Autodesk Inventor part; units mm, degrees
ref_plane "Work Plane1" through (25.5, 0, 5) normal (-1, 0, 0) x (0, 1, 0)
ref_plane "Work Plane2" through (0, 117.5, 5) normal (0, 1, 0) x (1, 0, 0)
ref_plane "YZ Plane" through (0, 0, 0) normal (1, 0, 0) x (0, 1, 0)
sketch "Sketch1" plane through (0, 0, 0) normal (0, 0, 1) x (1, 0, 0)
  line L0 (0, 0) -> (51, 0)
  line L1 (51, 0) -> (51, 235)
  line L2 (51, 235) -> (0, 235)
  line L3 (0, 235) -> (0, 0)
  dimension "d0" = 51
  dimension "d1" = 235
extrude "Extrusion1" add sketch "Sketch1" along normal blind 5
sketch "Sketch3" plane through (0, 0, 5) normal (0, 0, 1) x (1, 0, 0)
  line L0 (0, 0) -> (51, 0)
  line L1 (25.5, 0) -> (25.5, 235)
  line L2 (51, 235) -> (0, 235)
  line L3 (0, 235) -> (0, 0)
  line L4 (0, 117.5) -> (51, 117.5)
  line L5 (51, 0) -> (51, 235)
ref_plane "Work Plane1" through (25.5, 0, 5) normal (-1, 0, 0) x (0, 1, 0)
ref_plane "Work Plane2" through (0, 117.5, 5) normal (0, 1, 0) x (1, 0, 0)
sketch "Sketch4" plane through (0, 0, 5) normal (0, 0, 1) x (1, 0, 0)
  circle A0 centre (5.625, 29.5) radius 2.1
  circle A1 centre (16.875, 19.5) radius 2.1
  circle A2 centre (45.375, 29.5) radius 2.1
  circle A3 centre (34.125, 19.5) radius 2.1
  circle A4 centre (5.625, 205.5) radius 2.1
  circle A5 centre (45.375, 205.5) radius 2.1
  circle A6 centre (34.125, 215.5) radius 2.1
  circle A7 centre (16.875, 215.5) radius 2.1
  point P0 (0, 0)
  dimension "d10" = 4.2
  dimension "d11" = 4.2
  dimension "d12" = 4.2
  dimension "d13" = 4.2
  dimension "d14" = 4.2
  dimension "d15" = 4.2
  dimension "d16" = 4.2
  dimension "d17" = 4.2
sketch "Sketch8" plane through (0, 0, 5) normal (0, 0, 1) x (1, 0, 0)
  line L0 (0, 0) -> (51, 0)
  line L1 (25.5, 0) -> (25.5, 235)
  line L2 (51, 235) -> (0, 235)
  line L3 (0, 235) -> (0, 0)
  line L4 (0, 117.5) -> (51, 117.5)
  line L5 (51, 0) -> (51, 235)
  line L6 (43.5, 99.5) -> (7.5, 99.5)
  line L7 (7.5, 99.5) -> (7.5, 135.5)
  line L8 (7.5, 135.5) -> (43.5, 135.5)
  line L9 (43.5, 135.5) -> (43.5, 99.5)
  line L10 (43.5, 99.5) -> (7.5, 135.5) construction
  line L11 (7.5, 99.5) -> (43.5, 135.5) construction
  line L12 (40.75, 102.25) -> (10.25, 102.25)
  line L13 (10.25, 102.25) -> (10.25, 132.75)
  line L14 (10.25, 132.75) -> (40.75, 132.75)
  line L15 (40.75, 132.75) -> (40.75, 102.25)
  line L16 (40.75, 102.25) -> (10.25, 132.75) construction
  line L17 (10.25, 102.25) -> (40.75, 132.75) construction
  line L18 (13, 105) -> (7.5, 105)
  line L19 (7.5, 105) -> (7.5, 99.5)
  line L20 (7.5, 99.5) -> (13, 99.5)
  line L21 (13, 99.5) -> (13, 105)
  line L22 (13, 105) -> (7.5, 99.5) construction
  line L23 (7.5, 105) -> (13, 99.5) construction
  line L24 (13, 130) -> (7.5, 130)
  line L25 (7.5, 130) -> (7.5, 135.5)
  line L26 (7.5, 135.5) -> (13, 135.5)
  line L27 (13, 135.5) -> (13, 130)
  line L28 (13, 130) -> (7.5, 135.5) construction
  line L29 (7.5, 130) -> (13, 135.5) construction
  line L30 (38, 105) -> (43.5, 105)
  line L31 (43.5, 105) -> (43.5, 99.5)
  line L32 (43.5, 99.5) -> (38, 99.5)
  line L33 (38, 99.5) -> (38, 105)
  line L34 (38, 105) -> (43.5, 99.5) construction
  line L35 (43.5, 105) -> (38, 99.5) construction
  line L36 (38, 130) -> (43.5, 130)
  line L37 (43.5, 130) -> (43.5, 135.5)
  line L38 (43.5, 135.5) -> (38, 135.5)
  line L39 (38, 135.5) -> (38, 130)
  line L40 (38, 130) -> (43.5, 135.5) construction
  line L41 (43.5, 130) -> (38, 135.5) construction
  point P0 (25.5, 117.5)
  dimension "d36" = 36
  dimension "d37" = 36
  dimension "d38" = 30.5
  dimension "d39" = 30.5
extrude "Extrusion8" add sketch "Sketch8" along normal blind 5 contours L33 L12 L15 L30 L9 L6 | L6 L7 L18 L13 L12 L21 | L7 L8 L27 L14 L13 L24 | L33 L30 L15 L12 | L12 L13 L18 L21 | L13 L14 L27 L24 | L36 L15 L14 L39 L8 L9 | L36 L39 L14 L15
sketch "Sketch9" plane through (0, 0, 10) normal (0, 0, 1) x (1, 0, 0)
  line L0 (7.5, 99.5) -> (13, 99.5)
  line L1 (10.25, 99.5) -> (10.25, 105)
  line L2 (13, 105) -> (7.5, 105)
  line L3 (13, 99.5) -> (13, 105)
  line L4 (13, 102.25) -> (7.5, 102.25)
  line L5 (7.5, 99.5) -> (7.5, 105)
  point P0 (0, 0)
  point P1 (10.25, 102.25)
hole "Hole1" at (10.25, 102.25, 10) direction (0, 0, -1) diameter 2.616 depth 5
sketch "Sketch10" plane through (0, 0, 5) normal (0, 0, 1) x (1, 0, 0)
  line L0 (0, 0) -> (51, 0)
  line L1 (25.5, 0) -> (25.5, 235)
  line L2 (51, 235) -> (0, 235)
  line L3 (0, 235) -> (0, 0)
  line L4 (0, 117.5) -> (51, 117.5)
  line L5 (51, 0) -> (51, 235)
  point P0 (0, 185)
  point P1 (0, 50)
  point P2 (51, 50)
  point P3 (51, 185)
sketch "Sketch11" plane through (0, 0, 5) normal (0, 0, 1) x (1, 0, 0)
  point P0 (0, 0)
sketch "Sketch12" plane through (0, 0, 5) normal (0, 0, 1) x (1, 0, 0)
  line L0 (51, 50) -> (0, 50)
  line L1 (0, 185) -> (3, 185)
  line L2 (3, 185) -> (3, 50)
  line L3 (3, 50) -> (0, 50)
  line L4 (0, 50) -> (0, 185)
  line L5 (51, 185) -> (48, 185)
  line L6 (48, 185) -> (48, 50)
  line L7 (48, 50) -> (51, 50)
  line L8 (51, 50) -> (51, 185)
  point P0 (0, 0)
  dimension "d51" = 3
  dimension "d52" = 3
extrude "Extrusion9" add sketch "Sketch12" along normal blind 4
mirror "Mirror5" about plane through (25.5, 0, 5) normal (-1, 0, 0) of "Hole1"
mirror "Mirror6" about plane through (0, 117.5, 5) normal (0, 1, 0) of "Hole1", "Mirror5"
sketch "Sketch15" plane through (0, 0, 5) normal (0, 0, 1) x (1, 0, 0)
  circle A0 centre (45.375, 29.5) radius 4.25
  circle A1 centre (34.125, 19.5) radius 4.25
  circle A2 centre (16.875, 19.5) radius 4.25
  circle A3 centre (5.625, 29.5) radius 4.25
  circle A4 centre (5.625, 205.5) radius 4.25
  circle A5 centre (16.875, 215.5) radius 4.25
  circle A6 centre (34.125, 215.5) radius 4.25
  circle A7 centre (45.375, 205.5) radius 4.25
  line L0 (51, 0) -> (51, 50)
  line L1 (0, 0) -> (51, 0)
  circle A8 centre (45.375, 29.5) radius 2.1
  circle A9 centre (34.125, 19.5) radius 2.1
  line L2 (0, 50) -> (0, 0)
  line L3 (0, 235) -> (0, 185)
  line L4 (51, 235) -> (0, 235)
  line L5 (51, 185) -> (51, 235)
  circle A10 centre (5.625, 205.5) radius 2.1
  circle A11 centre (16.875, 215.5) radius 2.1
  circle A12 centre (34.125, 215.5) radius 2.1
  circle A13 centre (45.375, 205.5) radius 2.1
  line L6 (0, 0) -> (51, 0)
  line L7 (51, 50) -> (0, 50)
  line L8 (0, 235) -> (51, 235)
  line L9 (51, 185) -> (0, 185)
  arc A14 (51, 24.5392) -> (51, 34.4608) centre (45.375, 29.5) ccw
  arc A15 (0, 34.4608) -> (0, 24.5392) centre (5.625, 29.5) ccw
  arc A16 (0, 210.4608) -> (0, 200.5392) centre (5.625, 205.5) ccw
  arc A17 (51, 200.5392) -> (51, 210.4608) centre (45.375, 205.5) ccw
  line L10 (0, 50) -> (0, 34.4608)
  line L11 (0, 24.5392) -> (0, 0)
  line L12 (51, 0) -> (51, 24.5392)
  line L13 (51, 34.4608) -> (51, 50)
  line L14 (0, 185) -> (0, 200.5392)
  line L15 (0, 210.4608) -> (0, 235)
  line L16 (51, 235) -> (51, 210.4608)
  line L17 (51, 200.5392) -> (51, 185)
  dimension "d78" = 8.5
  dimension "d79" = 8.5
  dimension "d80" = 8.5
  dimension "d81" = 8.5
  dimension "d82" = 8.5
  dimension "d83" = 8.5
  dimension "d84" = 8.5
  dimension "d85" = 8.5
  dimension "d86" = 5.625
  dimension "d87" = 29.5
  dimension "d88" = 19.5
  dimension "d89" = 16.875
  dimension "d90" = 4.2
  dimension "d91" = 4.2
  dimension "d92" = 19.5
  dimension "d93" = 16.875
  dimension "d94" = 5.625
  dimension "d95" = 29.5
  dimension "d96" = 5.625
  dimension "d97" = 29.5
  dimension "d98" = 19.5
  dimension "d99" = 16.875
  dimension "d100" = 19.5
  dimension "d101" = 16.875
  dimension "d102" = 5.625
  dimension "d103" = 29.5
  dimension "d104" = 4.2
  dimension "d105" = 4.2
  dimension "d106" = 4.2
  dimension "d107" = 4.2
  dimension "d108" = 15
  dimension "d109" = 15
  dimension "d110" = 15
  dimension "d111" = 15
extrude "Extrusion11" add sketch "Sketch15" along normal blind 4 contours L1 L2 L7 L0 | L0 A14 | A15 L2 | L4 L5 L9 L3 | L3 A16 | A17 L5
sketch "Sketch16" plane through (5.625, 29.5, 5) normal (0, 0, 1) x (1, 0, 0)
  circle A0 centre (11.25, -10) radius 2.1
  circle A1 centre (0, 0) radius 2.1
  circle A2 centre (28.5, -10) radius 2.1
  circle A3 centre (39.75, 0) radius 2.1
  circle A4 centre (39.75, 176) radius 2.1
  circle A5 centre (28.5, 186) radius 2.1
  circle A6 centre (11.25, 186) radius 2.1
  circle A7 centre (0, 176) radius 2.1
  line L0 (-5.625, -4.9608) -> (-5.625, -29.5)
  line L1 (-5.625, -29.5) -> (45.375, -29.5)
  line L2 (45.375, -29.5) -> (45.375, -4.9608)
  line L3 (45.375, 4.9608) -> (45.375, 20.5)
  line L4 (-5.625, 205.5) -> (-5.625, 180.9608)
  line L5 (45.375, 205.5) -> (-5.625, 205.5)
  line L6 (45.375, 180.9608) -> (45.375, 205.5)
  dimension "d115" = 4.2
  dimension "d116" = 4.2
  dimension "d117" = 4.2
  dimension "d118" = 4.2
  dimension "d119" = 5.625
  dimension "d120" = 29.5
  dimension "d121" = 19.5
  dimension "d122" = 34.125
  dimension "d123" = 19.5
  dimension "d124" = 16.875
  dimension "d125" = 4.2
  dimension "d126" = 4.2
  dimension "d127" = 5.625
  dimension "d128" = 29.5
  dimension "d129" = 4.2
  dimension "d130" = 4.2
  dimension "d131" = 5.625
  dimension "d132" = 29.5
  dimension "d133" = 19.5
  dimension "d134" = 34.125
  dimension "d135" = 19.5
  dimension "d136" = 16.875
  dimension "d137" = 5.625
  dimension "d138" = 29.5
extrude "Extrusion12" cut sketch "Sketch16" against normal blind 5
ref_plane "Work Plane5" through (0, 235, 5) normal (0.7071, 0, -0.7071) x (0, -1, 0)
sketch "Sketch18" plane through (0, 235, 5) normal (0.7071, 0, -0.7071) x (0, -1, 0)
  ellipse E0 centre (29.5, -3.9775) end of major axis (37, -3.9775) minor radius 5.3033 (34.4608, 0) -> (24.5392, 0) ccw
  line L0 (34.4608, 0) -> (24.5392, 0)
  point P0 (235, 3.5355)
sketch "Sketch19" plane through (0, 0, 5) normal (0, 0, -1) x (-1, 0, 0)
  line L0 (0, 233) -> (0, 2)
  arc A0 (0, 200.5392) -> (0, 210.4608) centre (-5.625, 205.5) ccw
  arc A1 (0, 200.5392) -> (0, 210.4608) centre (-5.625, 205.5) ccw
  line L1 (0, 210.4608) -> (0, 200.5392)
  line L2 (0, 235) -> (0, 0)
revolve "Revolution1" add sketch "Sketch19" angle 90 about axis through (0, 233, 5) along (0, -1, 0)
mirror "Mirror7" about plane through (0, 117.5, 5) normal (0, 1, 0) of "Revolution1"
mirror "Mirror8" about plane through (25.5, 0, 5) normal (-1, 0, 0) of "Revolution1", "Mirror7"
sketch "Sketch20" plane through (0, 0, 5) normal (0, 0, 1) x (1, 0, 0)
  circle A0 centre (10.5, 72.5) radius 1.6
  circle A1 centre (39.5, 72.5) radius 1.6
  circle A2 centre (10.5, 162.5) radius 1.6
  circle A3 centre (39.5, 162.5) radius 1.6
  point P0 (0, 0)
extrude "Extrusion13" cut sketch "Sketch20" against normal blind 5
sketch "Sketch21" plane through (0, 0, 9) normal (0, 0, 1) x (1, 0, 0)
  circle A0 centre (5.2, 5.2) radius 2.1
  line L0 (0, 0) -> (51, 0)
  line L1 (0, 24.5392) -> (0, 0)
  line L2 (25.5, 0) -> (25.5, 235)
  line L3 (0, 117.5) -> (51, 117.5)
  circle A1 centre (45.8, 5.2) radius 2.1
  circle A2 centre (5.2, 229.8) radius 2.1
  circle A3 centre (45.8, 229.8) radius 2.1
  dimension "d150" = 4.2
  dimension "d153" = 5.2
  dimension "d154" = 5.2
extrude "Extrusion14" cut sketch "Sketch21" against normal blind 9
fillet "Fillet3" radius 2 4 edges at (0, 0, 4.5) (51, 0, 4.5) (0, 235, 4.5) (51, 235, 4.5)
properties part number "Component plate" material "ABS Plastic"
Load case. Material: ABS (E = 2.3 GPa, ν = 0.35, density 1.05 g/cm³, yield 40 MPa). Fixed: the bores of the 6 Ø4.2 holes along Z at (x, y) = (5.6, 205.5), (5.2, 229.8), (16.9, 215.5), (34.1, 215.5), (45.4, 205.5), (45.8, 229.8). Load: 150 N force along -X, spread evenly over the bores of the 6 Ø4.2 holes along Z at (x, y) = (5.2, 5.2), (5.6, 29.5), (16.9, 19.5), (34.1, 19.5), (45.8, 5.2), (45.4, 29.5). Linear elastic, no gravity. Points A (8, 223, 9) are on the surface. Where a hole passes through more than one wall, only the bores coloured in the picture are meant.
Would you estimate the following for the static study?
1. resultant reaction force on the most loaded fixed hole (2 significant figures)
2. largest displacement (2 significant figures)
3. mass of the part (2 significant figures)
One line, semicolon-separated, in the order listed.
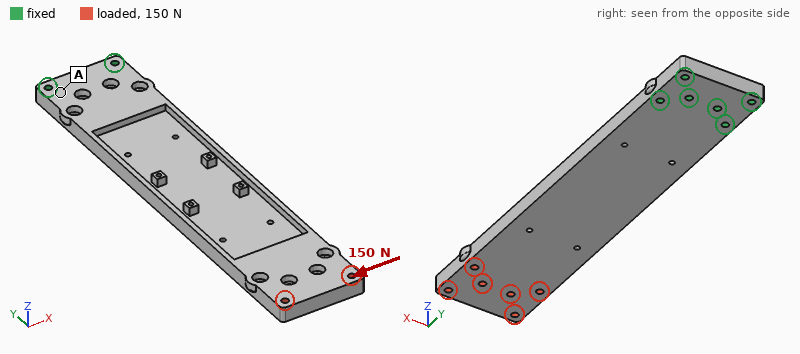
570 N; 2.7 mm; 85 g
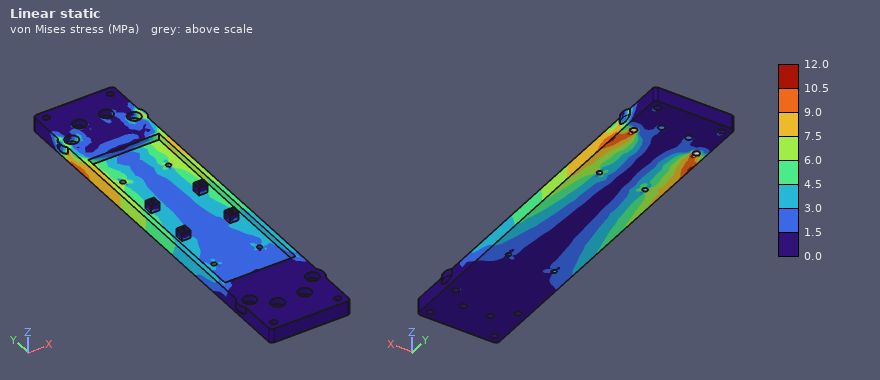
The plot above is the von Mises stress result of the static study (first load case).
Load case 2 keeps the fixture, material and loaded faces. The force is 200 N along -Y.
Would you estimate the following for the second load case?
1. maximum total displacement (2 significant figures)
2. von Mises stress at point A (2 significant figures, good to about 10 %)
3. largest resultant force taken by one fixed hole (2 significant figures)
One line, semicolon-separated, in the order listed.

0.71 mm; 0.14 MPa; 58 N
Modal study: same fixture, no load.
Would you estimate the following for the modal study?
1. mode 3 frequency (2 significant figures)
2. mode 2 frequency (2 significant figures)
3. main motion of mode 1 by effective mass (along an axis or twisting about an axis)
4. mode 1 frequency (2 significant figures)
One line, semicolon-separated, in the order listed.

240 Hz; 200 Hz; along Z; 35 Hz
